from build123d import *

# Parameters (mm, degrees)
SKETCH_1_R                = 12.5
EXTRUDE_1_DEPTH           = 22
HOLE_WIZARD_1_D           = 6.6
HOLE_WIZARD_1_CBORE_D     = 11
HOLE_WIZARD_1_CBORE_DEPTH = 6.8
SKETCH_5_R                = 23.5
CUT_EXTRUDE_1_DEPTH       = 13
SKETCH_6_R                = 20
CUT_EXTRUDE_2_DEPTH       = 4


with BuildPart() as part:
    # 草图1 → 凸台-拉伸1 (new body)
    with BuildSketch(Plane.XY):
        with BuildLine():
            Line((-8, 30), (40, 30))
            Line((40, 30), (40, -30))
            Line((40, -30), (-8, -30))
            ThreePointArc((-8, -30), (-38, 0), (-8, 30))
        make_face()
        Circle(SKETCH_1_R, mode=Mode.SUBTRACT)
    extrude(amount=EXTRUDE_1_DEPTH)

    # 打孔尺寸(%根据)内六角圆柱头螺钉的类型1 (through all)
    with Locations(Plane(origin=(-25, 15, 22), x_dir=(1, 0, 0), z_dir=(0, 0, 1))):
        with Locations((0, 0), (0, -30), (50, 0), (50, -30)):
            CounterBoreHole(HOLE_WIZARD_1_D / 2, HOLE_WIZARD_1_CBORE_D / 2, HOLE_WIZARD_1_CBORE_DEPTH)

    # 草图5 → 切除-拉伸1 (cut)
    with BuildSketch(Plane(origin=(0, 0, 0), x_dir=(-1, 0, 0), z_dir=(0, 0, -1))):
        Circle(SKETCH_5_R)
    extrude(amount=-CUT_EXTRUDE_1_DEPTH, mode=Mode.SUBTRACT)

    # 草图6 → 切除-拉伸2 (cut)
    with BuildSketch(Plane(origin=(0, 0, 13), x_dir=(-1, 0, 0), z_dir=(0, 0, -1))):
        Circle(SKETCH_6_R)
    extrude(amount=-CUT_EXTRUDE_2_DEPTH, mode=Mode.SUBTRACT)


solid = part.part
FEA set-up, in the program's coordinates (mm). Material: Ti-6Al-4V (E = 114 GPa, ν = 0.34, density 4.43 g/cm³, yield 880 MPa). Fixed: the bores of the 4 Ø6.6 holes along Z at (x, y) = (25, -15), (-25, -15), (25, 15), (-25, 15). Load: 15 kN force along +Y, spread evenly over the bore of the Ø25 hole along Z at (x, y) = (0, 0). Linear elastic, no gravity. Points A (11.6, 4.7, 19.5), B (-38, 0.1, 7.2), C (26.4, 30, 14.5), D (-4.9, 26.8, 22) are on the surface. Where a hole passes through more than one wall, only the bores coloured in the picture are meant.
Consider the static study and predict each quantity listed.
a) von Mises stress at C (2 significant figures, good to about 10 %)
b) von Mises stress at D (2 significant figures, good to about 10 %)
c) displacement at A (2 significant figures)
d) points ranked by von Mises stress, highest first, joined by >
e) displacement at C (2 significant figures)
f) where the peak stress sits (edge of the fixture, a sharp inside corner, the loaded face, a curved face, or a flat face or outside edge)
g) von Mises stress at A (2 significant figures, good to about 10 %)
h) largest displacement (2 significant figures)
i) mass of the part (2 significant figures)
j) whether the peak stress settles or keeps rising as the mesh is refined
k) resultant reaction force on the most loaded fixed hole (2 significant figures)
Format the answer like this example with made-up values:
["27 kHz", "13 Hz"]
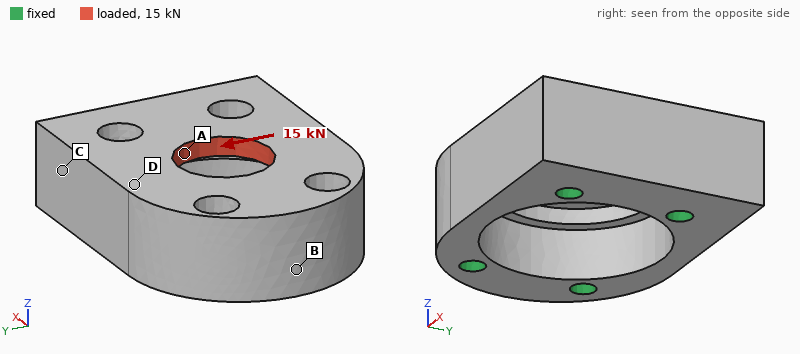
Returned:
["16 MPa", "26 MPa", "12 µm", "A > D > C > B", "4.1 µm", "edge of the fixture", "70 MPa", "18 µm", "260 g", "keeps rising", "4.1 kN"]
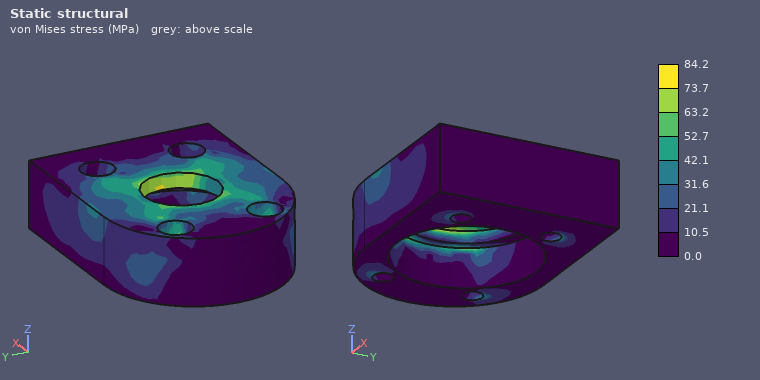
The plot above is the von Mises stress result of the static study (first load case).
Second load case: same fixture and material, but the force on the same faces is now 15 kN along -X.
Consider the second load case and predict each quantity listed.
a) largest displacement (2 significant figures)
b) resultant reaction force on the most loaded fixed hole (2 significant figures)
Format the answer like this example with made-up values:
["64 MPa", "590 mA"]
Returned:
["15 µm", "4.0 kN"]
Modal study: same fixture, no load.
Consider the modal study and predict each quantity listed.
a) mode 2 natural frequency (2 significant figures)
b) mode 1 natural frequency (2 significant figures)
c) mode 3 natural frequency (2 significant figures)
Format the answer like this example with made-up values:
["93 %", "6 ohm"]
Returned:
["20 kHz", "20 kHz", "24 kHz"]
